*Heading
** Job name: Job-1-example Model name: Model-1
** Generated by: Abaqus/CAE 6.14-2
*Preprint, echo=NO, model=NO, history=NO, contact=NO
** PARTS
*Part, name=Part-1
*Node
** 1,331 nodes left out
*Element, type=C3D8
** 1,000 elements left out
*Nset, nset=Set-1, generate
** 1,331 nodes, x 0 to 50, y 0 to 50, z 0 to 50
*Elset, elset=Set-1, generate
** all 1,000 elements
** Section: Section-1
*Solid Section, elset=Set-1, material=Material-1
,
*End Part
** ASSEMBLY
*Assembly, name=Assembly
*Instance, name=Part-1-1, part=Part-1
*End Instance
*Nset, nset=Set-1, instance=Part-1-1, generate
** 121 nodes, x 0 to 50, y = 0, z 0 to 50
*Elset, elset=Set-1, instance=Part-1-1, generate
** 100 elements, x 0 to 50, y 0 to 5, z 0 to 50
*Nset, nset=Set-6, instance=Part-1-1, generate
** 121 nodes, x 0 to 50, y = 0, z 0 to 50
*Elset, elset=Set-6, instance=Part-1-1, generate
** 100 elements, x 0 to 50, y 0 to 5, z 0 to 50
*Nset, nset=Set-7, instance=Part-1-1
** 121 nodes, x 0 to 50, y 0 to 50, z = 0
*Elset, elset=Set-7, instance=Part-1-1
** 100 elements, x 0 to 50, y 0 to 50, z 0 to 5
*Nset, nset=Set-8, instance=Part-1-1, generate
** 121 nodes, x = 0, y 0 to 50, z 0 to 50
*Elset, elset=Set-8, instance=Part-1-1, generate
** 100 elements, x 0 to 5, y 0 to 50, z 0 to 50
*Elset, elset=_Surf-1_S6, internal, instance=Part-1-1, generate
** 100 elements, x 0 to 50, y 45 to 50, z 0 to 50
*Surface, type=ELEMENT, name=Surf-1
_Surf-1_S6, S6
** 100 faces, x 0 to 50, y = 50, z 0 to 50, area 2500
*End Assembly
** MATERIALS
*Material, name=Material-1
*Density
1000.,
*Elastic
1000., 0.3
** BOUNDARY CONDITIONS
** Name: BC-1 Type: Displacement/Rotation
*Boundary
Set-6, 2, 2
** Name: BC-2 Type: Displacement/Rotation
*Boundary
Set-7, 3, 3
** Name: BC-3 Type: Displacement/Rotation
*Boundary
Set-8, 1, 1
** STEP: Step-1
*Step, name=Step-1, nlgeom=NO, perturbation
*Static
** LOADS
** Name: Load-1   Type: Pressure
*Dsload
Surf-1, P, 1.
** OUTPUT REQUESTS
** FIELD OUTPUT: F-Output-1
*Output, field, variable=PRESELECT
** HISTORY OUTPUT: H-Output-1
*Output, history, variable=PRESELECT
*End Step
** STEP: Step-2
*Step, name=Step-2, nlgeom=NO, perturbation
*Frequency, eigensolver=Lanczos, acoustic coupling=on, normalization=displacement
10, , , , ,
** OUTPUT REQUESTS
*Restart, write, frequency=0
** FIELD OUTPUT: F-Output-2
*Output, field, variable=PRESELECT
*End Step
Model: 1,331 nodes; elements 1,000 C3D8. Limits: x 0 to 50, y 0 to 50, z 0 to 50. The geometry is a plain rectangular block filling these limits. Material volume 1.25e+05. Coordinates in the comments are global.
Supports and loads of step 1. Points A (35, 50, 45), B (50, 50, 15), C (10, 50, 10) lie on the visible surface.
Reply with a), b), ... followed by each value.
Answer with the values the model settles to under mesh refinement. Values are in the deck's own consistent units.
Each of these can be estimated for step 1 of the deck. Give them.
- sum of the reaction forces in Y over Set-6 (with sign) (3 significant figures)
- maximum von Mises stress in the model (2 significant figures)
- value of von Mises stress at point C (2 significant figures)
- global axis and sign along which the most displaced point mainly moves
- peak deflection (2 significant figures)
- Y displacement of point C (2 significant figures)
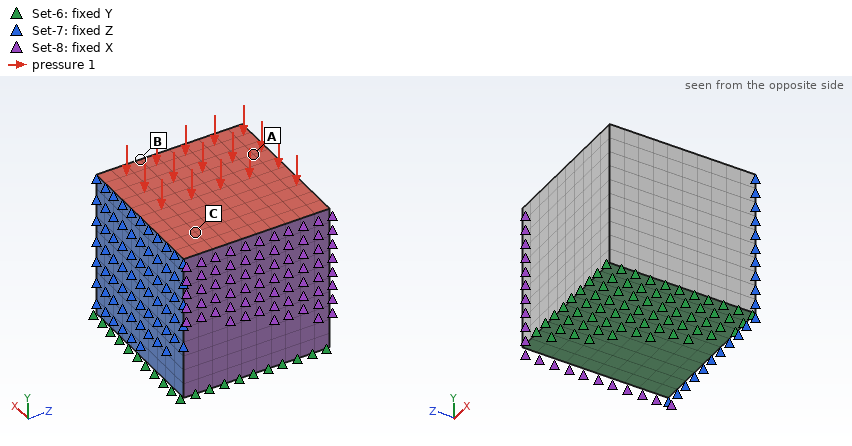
a) 2500
b) 1.0
c) 1.0
d) -Y
e) 0.054
f) -0.050
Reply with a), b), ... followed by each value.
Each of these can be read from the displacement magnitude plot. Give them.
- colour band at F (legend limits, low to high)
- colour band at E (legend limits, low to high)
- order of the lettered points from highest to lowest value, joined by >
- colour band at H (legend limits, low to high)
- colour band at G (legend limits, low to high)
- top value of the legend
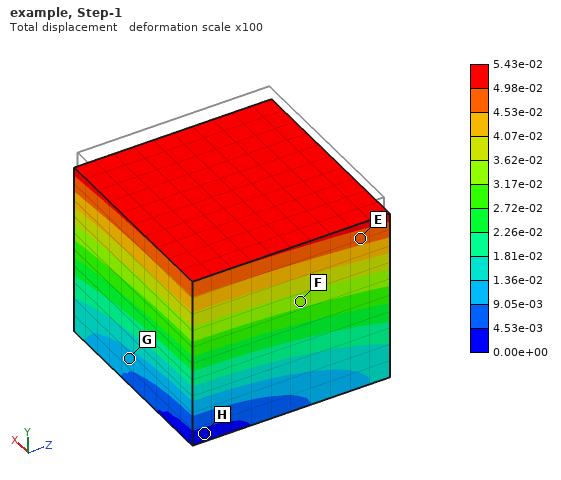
a) 3.17e-02 to 3.62e-02
b) 4.53e-02 to 4.98e-02
c) E > F > G > H
d) 0.00e+00 to 4.53e-03
e) 9.05e-03 to 1.36e-02
f) 5.43e-02
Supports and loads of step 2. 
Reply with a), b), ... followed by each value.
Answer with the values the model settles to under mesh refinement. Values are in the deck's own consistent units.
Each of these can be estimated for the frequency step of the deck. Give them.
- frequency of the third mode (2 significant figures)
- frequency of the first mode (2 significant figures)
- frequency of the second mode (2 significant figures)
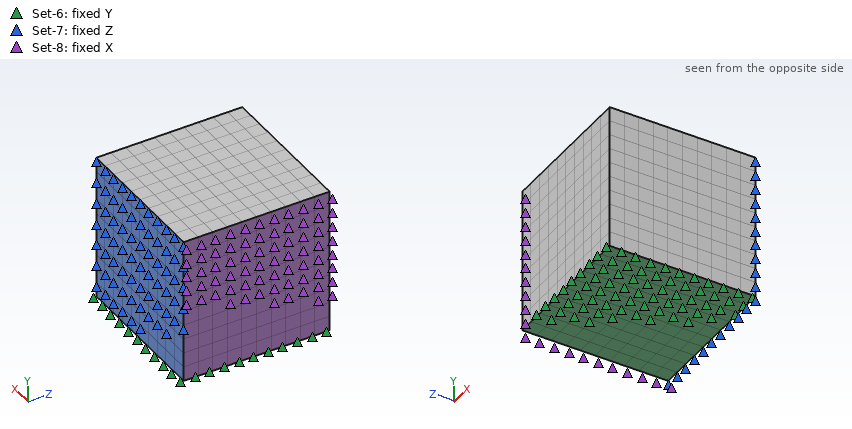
a) 0.16 cycles per unit time
b) 0.16 cycles per unit time
c) 0.16 cycles per unit time
